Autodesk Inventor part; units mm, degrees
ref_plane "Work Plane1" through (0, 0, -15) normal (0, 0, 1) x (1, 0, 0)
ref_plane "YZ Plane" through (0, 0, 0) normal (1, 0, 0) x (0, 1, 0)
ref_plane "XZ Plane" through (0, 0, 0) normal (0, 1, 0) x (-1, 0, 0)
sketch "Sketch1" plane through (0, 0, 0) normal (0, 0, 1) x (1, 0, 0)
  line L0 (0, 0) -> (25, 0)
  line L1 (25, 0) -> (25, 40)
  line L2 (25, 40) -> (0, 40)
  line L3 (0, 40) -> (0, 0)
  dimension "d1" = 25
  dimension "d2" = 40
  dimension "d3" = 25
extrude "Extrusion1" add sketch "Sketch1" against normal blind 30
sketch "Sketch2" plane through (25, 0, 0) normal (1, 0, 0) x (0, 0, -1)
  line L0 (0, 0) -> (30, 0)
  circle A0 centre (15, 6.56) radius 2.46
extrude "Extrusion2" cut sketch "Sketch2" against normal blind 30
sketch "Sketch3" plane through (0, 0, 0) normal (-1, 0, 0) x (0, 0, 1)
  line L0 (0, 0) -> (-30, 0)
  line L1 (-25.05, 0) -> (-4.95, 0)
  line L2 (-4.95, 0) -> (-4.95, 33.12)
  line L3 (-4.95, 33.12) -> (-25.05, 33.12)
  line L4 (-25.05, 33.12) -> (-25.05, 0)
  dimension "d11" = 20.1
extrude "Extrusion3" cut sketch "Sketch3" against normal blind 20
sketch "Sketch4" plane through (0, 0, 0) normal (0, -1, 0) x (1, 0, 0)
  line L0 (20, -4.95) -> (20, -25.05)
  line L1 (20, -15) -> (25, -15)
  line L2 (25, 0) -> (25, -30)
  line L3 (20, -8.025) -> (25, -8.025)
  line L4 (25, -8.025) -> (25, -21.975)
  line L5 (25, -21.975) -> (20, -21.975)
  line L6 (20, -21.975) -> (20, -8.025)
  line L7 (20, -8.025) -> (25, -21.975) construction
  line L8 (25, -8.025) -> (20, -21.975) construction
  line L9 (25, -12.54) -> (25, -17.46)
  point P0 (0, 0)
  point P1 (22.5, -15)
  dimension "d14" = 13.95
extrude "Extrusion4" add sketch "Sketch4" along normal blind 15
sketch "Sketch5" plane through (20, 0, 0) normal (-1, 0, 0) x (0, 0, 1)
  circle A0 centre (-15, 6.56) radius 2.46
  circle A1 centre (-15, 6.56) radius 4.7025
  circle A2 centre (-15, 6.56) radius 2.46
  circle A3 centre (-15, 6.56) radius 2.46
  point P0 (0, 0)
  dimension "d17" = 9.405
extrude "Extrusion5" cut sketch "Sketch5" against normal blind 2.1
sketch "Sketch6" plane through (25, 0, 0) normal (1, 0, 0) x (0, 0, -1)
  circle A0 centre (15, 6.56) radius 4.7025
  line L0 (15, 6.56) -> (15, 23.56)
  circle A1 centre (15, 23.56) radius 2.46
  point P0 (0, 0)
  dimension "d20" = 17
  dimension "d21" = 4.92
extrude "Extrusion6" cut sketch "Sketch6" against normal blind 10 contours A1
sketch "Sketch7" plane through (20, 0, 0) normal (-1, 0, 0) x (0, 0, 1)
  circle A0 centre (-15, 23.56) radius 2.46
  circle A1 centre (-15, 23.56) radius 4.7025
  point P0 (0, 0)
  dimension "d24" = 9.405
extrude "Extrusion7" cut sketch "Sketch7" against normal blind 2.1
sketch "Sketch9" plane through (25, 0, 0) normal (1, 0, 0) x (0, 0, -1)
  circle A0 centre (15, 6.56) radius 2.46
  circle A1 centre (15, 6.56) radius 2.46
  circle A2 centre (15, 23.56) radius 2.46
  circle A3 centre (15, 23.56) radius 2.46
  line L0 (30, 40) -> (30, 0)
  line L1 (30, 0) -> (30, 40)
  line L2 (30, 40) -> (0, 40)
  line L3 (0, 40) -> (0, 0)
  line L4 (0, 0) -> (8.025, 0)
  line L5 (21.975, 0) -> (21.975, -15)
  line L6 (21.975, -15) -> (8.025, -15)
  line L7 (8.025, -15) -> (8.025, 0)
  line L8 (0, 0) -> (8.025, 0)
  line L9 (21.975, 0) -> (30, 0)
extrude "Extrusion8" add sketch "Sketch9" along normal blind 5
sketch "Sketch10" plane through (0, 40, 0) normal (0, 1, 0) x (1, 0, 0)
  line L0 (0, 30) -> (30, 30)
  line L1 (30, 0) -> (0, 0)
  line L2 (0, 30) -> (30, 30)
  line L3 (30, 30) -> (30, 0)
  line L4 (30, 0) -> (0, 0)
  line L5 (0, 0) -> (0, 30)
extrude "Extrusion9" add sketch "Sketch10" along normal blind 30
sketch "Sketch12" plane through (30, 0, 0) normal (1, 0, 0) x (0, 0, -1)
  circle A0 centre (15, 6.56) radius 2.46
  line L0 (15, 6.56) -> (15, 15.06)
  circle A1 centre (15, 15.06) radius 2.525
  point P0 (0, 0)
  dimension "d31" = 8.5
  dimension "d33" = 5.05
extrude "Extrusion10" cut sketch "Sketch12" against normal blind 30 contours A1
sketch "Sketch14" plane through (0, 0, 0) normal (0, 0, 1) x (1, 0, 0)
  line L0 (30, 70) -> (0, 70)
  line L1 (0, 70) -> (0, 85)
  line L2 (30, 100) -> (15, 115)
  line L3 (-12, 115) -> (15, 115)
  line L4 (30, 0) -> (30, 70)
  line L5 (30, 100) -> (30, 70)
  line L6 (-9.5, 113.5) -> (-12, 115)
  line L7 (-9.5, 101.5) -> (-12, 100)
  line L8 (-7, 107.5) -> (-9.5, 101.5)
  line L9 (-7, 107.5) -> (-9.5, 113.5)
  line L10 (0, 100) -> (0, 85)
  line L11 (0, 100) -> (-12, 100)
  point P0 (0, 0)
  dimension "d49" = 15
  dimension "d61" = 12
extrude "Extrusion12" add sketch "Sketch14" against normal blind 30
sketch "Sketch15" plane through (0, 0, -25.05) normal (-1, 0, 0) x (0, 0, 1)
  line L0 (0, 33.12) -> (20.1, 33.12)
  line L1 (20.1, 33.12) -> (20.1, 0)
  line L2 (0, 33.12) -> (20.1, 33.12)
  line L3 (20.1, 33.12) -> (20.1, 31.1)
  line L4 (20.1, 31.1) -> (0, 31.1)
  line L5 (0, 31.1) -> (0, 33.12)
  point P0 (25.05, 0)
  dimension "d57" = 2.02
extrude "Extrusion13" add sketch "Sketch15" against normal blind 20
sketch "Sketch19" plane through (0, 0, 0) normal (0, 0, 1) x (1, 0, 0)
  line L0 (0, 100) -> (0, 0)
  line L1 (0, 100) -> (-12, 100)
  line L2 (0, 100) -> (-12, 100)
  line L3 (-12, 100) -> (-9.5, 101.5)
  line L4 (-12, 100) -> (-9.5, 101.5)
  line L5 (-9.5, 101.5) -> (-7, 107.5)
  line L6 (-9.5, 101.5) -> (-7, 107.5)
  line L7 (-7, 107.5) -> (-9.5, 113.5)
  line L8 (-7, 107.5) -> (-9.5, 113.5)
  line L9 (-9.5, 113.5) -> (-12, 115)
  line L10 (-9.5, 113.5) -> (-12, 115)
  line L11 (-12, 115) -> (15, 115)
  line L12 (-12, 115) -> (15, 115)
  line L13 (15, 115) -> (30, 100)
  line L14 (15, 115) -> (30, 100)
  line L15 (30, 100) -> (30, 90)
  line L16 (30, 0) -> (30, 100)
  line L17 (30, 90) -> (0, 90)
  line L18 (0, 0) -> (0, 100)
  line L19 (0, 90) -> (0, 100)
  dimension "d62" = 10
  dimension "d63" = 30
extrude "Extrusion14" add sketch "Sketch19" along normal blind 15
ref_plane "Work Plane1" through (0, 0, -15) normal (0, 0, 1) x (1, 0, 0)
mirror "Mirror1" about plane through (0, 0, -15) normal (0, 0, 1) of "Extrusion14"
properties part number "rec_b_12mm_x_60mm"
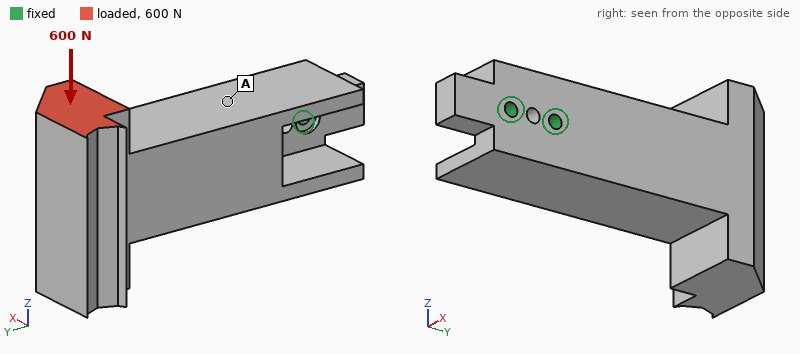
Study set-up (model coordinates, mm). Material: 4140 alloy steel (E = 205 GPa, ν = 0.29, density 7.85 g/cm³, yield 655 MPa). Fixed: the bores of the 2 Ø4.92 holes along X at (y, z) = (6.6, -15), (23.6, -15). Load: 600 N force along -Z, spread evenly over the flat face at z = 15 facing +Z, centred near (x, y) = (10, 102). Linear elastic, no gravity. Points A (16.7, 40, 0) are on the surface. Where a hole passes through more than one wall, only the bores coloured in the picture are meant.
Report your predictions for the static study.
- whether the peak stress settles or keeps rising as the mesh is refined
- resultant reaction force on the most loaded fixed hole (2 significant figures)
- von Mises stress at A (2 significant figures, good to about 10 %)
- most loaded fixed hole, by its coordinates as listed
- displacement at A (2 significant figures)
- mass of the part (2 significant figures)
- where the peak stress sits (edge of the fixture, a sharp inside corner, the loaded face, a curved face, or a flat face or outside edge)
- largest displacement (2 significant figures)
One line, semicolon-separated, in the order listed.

keeps rising; 2.6 kN; 10.0 MPa; (23.6, -15); 6.2 µm; 910 g; edge of the fixture; 33 µm
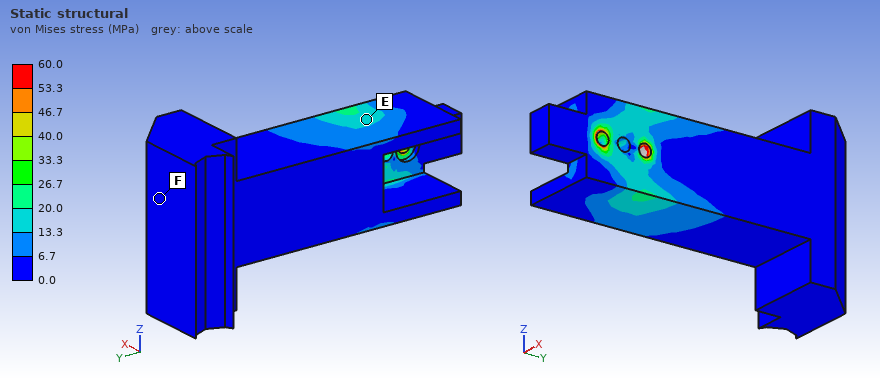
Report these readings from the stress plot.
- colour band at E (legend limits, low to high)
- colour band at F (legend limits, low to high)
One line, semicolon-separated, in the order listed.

13.3 to 20.0 MPa; 0.0 to 6.7 MPa
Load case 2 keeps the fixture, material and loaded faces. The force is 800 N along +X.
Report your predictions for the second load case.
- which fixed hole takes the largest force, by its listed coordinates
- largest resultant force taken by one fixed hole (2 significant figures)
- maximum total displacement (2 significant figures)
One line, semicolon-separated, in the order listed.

(23.6, -15); 3.3 kN; 75 µm
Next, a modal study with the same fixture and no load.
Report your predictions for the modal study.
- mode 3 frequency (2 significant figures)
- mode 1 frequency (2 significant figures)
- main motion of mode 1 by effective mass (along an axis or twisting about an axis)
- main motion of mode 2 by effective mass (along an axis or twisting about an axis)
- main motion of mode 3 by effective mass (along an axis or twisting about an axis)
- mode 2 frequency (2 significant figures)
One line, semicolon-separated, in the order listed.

2400 Hz; 950 Hz; along X; along Z; twisting about Y; 1100 Hz
